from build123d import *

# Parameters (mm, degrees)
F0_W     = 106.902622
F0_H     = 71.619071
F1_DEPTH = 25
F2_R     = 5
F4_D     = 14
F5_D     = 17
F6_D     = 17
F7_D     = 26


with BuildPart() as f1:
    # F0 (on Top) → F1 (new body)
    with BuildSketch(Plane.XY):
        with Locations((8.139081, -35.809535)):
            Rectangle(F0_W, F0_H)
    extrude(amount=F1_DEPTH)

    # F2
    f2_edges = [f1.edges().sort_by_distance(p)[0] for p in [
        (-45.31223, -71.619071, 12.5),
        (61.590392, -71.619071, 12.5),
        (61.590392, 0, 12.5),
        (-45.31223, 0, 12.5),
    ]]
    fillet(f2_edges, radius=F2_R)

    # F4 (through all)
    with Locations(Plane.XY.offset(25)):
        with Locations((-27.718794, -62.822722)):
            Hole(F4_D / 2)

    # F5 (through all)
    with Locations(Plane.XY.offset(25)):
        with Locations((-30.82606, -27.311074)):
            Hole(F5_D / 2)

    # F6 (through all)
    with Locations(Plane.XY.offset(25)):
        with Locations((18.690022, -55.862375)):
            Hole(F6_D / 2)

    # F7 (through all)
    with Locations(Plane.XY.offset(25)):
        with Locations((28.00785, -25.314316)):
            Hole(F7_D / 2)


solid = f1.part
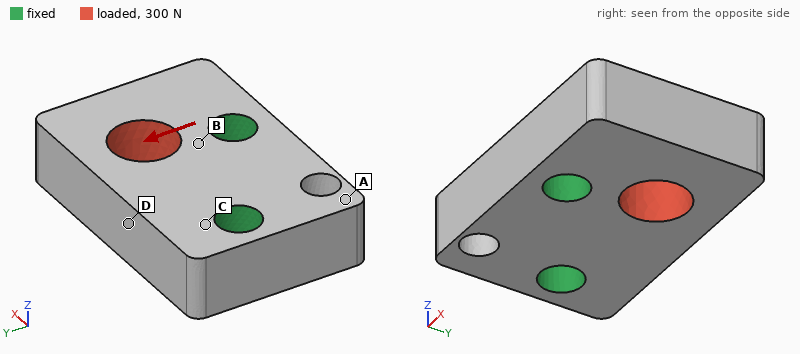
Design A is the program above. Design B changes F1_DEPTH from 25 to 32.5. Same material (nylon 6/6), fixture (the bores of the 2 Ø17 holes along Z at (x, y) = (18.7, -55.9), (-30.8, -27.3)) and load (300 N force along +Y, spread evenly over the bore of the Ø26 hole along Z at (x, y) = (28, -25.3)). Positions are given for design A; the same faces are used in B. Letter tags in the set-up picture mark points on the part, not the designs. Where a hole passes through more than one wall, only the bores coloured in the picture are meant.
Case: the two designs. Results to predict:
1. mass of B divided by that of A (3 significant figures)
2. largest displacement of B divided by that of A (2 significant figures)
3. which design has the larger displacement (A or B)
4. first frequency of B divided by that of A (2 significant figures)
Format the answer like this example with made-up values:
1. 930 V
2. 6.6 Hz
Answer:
1. 1.30
2. 0.75
3. A
4. 1.2
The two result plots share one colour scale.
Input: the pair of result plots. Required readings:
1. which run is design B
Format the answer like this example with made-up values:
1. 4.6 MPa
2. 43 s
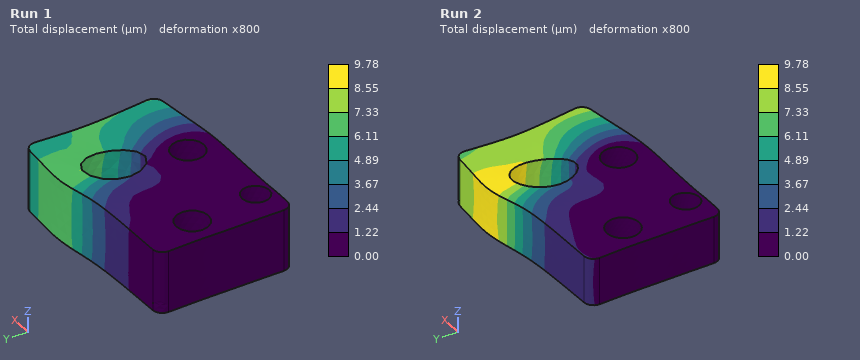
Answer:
1. Run 1
